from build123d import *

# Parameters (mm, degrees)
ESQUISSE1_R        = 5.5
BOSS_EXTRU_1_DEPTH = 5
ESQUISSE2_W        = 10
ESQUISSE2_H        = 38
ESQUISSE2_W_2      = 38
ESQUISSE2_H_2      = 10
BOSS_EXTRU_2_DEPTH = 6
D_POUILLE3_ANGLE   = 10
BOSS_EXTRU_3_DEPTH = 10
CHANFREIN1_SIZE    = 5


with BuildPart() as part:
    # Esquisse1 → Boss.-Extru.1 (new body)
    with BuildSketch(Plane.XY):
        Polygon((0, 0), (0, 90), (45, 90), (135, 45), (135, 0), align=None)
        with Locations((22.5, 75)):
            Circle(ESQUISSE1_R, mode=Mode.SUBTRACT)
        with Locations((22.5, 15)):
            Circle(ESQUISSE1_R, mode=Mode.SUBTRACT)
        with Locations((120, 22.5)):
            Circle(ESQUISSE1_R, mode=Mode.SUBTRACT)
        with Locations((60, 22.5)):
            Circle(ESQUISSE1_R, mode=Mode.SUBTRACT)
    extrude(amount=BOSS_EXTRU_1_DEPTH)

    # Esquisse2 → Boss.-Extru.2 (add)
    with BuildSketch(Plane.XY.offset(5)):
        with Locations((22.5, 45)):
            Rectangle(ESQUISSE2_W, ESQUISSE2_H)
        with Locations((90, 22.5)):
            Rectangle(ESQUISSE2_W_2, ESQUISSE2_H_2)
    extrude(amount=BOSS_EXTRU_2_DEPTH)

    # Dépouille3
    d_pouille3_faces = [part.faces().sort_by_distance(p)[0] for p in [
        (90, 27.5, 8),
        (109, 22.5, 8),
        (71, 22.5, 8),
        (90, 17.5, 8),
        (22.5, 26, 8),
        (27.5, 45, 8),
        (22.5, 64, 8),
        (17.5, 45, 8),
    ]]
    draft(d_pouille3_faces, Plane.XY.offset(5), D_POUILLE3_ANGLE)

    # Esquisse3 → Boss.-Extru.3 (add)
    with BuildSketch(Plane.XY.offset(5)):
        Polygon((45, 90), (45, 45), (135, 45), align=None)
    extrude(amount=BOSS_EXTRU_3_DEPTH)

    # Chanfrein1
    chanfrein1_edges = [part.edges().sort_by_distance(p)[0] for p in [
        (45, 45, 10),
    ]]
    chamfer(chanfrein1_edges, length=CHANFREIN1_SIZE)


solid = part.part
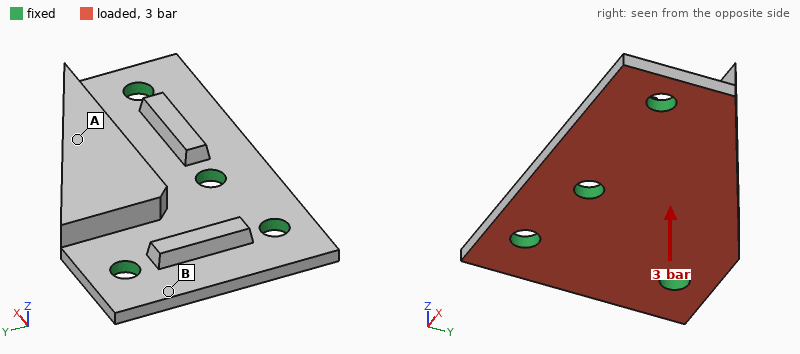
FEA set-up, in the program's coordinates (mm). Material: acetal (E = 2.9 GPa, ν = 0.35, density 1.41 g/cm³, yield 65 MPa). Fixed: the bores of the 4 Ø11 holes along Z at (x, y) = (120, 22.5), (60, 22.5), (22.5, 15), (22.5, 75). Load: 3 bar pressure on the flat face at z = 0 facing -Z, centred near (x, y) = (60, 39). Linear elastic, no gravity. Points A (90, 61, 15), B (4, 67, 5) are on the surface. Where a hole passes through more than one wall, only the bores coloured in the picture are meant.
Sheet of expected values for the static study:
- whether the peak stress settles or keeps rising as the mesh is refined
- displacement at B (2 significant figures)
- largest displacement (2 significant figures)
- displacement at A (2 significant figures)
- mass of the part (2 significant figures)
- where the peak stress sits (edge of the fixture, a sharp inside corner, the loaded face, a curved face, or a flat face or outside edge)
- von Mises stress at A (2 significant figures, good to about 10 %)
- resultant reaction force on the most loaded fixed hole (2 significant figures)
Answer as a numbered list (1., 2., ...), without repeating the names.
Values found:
1. keeps rising
2. 0.17 mm
3. 0.96 mm
4. 0.85 mm
5. 100 g
6. edge of the fixture
7. 7.1 MPa
8. 960 N
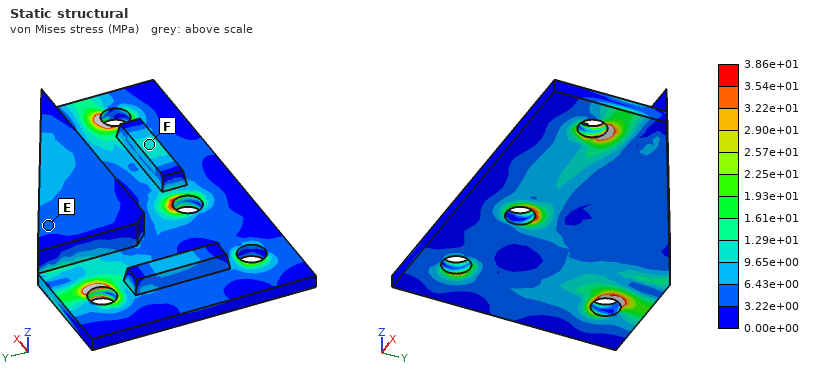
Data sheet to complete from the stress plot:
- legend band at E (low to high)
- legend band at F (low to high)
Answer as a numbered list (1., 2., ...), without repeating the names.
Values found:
1. 3.22e+00 to 6.43e+00 MPa
2. 9.65e+00 to 1.29e+01 MPa
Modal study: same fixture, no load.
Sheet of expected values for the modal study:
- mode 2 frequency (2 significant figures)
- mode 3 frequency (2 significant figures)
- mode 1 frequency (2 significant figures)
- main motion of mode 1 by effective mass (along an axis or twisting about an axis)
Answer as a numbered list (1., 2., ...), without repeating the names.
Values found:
1. 1800 Hz
2. 2200 Hz
3. 790 Hz
4. along Z
